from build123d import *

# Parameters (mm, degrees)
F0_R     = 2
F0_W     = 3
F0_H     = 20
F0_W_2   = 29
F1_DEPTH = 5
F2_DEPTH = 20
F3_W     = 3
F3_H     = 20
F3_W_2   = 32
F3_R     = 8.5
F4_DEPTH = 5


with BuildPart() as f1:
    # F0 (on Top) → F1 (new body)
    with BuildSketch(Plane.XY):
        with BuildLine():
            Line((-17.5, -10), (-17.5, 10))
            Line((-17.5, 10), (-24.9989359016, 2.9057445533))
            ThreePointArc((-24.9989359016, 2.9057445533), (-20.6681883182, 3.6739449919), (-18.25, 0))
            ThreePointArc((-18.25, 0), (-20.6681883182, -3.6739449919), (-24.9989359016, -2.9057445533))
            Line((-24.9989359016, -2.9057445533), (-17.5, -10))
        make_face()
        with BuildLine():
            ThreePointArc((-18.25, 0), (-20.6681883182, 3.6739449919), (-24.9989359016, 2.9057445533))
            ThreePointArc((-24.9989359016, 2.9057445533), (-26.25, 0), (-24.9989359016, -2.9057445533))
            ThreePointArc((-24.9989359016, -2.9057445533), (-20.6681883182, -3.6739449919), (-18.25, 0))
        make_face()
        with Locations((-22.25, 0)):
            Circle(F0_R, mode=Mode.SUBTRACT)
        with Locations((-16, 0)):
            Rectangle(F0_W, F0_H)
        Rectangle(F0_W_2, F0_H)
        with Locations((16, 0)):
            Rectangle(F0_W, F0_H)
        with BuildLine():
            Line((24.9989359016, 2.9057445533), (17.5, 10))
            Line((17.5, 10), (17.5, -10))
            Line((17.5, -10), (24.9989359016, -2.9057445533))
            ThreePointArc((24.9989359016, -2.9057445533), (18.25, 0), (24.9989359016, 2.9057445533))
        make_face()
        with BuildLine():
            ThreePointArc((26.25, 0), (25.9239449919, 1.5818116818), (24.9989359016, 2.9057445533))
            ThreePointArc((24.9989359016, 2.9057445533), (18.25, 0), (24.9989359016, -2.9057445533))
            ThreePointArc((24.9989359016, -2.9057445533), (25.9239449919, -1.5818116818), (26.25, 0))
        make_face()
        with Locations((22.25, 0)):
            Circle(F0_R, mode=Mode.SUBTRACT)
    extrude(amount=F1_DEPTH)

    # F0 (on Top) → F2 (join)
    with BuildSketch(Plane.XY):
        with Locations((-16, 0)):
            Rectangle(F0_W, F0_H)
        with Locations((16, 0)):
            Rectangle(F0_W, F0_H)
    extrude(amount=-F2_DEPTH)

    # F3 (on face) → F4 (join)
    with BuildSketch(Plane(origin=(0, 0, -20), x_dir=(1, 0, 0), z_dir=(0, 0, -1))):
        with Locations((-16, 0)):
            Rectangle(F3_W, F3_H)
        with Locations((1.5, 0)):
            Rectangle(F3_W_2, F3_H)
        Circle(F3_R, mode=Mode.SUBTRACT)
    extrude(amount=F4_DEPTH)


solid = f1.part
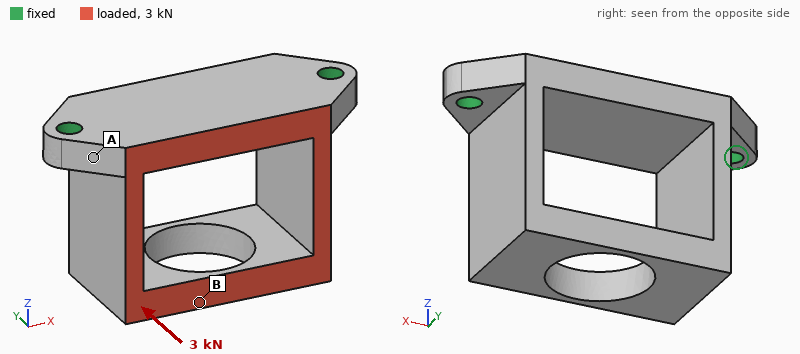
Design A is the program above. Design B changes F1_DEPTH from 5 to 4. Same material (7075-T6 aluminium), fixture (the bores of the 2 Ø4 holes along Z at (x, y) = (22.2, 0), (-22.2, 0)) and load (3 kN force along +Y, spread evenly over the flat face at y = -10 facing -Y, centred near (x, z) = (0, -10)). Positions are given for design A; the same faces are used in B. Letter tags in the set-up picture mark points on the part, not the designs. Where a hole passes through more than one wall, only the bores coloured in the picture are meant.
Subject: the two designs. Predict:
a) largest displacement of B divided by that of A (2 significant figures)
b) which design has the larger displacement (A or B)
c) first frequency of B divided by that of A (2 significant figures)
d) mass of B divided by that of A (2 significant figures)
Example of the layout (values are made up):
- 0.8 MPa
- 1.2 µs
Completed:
- 1.6
- B
- 0.91
- 0.90
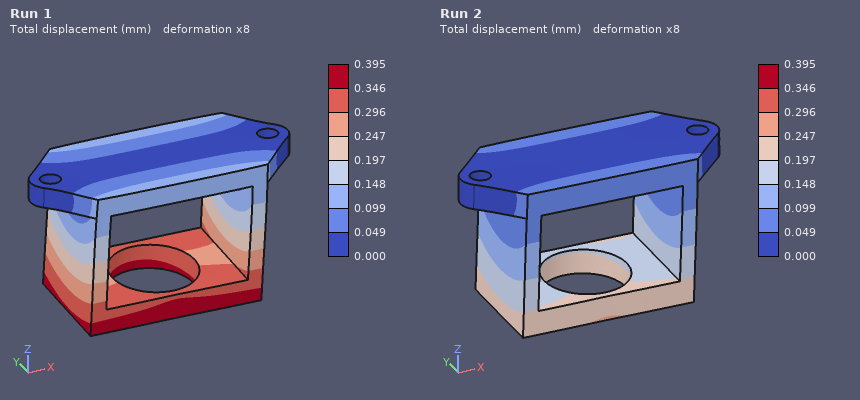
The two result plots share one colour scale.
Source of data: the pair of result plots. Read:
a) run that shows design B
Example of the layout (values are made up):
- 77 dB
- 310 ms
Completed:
- Run 1
